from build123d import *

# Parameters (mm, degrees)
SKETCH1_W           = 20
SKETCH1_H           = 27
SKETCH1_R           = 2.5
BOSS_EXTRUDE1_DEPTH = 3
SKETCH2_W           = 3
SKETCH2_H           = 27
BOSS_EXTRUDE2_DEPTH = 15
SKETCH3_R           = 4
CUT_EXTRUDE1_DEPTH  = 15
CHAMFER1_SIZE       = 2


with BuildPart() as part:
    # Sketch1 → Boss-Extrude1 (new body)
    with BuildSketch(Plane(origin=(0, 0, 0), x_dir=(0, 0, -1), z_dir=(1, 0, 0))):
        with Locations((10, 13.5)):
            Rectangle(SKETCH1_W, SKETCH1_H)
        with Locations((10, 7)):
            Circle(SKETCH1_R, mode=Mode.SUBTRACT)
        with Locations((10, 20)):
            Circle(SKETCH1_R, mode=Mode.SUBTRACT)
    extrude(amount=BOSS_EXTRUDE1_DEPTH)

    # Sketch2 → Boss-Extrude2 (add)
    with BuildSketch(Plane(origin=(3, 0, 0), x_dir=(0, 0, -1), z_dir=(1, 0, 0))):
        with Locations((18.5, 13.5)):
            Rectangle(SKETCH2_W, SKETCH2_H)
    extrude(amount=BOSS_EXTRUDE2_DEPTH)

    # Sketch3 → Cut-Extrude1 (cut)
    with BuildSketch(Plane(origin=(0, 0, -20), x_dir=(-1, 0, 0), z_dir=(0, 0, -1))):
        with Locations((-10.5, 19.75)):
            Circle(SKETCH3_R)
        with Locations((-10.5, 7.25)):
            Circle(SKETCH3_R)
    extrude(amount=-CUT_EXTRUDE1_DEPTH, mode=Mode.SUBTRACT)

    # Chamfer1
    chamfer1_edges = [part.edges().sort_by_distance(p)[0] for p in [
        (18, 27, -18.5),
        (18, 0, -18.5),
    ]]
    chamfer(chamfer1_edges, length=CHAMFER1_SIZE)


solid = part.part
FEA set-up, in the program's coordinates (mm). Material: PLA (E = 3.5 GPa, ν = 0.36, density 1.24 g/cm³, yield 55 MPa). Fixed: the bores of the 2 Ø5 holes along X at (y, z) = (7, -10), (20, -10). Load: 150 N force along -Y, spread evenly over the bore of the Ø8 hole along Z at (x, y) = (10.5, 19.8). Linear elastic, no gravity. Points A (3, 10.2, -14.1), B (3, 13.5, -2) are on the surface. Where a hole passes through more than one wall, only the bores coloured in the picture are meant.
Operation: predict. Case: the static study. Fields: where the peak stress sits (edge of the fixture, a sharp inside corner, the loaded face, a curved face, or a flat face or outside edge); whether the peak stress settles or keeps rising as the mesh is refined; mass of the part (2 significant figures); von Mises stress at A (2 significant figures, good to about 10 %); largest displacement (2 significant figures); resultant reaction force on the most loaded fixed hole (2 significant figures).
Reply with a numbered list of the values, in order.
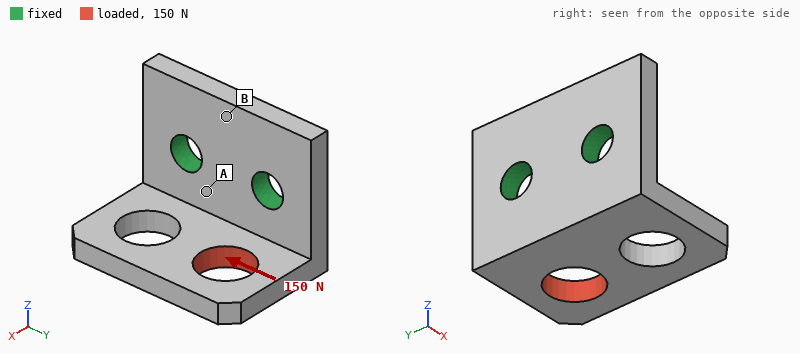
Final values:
1. edge of the fixture
2. keeps rising
3. 3.0 g
4. 11 MPa
5. 0.24 mm
6. 130 N
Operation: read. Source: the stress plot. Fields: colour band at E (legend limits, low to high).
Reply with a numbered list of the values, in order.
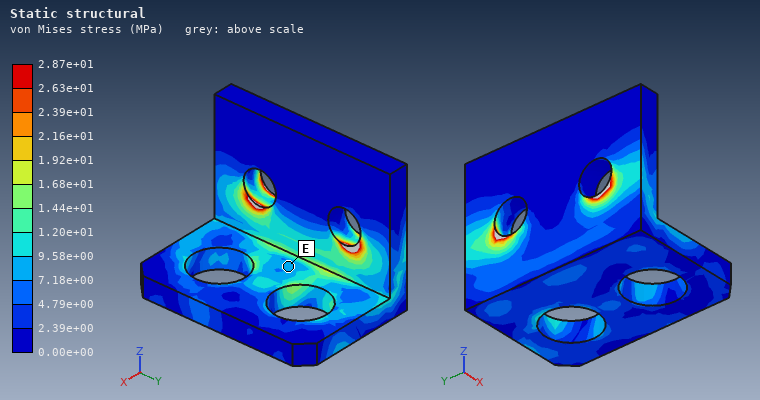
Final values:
1. 7.18e+00 to 9.58e+00 MPa
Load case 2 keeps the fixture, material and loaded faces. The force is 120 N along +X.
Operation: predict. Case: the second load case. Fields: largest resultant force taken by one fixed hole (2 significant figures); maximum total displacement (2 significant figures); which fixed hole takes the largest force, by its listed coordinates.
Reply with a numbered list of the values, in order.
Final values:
1. 100 N
2. 0.33 mm
3. (20, -10)
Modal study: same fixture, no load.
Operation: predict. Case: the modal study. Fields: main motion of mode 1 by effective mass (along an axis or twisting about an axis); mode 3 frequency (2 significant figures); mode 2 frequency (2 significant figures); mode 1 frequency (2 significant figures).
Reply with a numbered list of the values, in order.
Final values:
1. along Z
2. 4900 Hz
3. 3400 Hz
4. 2000 Hz
